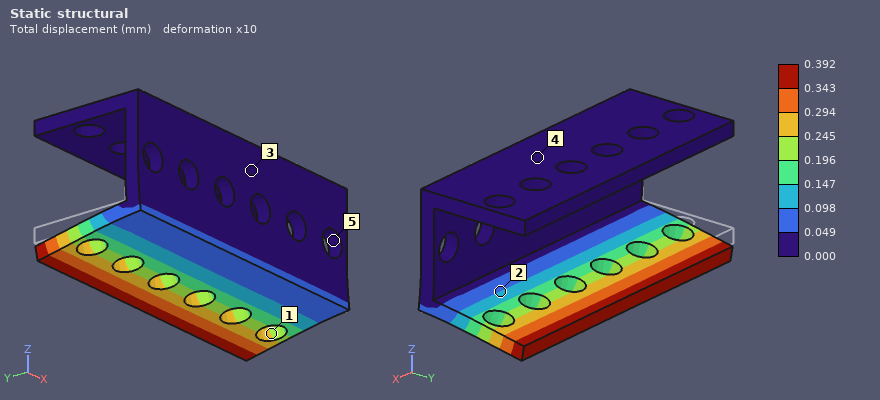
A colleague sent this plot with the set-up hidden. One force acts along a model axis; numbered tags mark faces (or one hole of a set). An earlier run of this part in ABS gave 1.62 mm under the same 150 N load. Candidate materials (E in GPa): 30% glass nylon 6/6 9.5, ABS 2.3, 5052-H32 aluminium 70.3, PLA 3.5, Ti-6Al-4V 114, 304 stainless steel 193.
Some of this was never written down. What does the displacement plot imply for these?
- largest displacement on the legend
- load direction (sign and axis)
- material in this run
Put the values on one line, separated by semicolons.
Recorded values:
0.392 mm; -Z; 30% glass nylon 6/6
